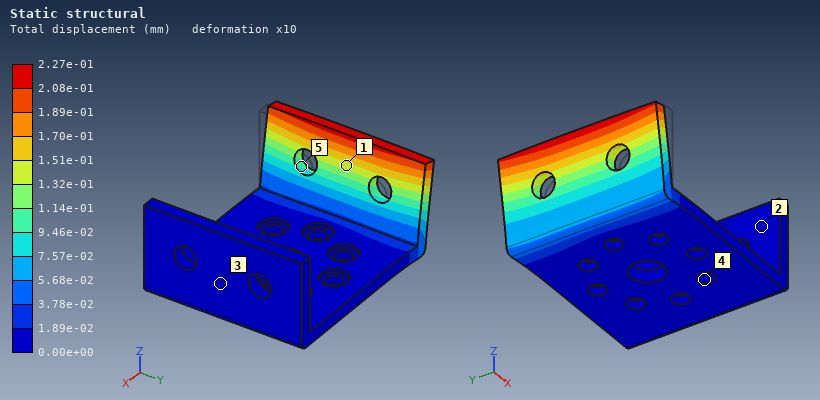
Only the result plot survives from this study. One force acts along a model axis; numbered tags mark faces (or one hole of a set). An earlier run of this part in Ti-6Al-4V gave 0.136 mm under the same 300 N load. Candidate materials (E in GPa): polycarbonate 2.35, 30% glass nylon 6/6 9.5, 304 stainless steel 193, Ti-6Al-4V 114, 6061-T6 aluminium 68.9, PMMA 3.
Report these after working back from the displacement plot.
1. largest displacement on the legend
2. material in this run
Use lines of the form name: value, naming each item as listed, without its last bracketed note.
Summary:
largest displacement on the legend: 2.27e-01 mm
material in this run: 6061-T6 aluminium
